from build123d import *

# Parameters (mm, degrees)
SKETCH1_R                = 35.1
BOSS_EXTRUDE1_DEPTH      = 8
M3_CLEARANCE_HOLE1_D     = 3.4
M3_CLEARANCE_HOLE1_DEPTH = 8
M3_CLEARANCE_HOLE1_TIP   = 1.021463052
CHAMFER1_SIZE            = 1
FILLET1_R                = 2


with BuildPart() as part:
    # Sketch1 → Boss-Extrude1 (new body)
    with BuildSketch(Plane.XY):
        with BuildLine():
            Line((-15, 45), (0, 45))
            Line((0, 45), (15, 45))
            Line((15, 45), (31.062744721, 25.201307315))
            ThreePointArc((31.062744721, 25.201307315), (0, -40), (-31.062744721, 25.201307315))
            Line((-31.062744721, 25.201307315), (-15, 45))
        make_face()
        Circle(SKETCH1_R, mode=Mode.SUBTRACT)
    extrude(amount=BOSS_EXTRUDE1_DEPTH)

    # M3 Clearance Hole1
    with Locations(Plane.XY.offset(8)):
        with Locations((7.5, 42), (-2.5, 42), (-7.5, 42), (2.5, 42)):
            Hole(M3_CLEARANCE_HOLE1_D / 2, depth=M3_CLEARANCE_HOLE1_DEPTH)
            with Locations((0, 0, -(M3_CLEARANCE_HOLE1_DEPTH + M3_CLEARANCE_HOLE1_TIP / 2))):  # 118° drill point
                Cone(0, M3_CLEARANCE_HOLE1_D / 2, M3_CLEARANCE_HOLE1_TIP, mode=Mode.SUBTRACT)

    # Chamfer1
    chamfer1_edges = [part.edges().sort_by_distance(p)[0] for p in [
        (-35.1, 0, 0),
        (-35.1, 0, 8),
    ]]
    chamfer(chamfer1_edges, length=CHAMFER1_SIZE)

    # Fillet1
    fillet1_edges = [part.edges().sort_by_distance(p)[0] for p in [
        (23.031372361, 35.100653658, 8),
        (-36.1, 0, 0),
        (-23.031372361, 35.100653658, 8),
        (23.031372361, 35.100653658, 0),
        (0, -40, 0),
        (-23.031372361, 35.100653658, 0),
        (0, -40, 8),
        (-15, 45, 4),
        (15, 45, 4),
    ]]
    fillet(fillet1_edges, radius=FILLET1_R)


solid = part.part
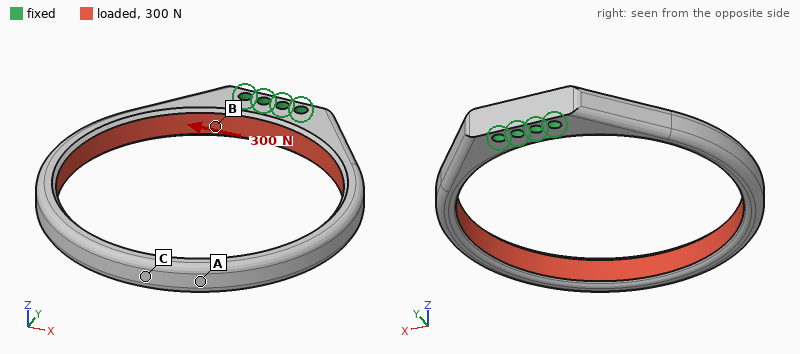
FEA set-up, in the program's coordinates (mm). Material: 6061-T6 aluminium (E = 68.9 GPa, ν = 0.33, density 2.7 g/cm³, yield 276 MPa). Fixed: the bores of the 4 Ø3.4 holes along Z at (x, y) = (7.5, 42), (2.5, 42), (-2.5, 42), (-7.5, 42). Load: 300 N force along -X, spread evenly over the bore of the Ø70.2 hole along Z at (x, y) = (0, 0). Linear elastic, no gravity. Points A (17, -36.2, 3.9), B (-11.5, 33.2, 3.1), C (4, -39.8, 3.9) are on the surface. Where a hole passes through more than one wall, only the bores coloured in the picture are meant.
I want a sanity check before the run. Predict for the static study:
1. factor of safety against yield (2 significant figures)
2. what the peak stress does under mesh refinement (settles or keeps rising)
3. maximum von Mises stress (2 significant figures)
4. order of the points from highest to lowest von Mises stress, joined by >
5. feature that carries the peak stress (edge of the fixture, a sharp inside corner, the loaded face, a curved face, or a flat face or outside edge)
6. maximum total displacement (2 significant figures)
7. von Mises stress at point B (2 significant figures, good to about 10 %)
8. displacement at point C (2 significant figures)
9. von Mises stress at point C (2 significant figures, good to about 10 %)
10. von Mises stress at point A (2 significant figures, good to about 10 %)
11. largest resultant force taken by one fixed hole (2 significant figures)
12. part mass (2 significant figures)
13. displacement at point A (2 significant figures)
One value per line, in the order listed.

2.9
settles
94 MPa
B > A > C
the loaded face
0.61 mm
42 MPa
0.61 mm
7.5 MPa
30 MPa
570 N
28 g
0.61 mm
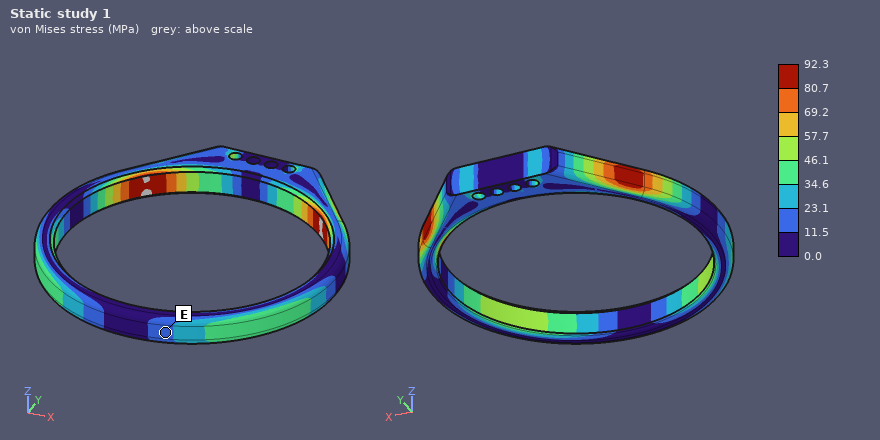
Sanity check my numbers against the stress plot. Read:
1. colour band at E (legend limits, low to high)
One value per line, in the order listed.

11.5 to 23.1 MPa
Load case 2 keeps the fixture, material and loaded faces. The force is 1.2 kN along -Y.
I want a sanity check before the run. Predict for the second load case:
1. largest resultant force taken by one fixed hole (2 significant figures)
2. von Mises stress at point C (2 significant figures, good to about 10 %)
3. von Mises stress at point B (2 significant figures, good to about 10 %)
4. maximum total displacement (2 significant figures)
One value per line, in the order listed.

1.5 kN
69 MPa
67 MPa
0.35 mm
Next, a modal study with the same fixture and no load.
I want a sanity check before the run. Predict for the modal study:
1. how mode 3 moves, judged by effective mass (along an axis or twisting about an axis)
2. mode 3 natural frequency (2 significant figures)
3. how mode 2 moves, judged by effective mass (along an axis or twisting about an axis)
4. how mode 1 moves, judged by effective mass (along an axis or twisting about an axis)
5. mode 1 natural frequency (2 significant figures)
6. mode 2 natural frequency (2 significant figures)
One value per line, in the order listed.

twisting about Y
1500 Hz
along X
along Z
610 Hz
790 Hz
